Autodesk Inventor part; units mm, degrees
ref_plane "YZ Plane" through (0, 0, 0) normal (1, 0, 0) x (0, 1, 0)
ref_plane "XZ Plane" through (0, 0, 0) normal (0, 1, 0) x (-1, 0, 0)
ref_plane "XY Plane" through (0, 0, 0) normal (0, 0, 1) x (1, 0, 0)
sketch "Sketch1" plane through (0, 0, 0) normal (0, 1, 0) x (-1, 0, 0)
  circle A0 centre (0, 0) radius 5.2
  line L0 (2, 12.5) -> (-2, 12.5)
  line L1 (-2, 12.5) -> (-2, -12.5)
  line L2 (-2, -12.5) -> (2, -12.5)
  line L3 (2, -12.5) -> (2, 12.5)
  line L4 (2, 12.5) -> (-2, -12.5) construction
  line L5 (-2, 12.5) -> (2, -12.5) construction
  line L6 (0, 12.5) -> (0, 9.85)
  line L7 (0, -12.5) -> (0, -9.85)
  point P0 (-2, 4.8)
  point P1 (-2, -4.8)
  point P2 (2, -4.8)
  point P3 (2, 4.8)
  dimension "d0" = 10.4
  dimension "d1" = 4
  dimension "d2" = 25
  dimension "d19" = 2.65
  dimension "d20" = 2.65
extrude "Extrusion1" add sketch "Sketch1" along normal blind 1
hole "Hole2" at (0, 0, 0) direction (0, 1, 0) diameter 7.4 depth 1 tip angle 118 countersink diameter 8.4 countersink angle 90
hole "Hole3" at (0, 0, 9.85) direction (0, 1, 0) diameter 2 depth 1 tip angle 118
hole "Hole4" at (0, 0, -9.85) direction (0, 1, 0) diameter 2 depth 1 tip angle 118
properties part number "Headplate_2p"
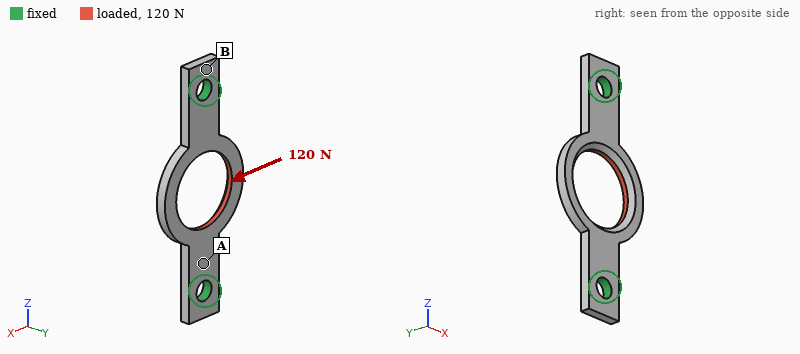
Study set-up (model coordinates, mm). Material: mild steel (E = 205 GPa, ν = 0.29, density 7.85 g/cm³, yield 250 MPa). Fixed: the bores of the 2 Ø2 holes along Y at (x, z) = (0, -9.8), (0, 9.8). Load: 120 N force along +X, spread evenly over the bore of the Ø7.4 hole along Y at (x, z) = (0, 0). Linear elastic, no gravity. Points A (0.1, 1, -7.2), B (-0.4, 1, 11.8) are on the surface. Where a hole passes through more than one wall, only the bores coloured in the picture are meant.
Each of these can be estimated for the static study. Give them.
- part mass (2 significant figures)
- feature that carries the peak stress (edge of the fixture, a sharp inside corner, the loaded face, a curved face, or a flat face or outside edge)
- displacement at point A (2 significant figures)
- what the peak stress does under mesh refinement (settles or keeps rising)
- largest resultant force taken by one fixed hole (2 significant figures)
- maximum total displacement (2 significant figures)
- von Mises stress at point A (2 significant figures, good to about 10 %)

0.72 g
edge of the fixture
1.2 µm
keeps rising
60 N
7.2 µm
59 MPa
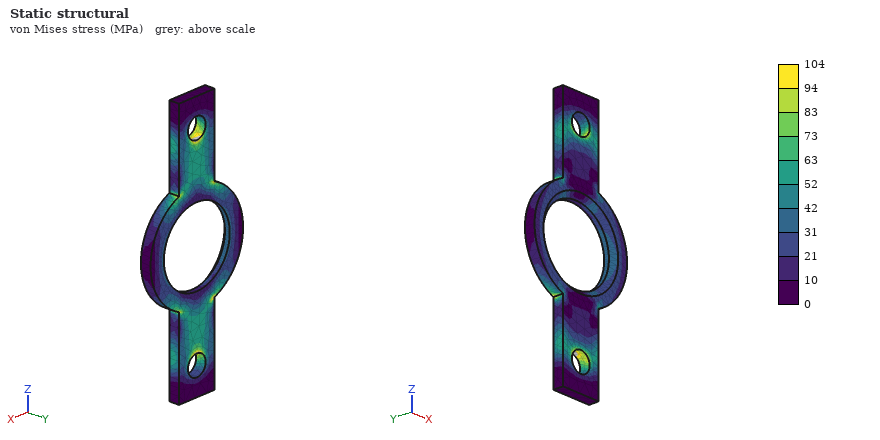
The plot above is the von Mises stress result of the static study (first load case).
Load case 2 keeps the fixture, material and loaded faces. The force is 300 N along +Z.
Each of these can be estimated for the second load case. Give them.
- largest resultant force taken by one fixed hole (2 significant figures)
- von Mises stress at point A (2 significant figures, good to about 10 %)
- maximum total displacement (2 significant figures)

150 N
42 MPa
3.9 µm
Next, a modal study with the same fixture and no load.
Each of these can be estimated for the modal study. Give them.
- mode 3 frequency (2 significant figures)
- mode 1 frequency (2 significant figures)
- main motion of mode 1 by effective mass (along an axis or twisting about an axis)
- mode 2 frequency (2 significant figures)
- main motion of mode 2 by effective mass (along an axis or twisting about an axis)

32 kHz
14 kHz
along Y
15 kHz
twisting about Z
